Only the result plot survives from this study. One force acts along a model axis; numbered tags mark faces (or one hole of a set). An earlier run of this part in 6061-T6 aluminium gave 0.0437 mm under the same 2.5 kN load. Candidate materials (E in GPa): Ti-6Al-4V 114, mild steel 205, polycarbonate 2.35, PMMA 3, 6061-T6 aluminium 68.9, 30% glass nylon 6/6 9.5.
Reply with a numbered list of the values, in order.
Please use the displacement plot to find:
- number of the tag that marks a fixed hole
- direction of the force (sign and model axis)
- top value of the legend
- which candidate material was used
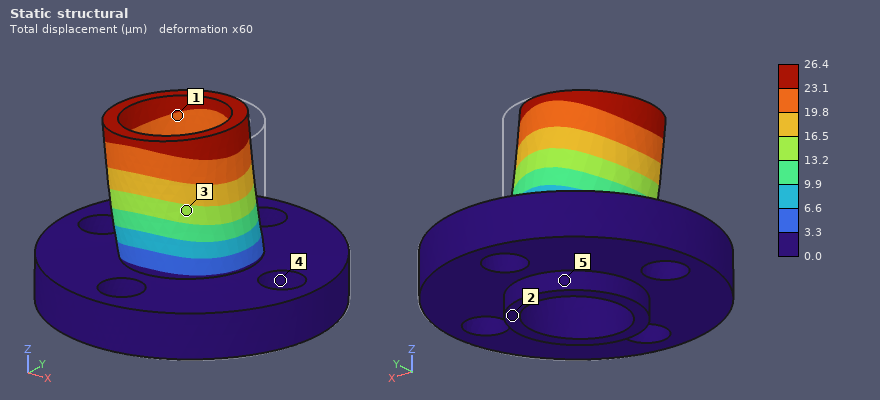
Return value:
1. 4
2. -X
3. 26.4 µm
4. Ti-6Al-4V
